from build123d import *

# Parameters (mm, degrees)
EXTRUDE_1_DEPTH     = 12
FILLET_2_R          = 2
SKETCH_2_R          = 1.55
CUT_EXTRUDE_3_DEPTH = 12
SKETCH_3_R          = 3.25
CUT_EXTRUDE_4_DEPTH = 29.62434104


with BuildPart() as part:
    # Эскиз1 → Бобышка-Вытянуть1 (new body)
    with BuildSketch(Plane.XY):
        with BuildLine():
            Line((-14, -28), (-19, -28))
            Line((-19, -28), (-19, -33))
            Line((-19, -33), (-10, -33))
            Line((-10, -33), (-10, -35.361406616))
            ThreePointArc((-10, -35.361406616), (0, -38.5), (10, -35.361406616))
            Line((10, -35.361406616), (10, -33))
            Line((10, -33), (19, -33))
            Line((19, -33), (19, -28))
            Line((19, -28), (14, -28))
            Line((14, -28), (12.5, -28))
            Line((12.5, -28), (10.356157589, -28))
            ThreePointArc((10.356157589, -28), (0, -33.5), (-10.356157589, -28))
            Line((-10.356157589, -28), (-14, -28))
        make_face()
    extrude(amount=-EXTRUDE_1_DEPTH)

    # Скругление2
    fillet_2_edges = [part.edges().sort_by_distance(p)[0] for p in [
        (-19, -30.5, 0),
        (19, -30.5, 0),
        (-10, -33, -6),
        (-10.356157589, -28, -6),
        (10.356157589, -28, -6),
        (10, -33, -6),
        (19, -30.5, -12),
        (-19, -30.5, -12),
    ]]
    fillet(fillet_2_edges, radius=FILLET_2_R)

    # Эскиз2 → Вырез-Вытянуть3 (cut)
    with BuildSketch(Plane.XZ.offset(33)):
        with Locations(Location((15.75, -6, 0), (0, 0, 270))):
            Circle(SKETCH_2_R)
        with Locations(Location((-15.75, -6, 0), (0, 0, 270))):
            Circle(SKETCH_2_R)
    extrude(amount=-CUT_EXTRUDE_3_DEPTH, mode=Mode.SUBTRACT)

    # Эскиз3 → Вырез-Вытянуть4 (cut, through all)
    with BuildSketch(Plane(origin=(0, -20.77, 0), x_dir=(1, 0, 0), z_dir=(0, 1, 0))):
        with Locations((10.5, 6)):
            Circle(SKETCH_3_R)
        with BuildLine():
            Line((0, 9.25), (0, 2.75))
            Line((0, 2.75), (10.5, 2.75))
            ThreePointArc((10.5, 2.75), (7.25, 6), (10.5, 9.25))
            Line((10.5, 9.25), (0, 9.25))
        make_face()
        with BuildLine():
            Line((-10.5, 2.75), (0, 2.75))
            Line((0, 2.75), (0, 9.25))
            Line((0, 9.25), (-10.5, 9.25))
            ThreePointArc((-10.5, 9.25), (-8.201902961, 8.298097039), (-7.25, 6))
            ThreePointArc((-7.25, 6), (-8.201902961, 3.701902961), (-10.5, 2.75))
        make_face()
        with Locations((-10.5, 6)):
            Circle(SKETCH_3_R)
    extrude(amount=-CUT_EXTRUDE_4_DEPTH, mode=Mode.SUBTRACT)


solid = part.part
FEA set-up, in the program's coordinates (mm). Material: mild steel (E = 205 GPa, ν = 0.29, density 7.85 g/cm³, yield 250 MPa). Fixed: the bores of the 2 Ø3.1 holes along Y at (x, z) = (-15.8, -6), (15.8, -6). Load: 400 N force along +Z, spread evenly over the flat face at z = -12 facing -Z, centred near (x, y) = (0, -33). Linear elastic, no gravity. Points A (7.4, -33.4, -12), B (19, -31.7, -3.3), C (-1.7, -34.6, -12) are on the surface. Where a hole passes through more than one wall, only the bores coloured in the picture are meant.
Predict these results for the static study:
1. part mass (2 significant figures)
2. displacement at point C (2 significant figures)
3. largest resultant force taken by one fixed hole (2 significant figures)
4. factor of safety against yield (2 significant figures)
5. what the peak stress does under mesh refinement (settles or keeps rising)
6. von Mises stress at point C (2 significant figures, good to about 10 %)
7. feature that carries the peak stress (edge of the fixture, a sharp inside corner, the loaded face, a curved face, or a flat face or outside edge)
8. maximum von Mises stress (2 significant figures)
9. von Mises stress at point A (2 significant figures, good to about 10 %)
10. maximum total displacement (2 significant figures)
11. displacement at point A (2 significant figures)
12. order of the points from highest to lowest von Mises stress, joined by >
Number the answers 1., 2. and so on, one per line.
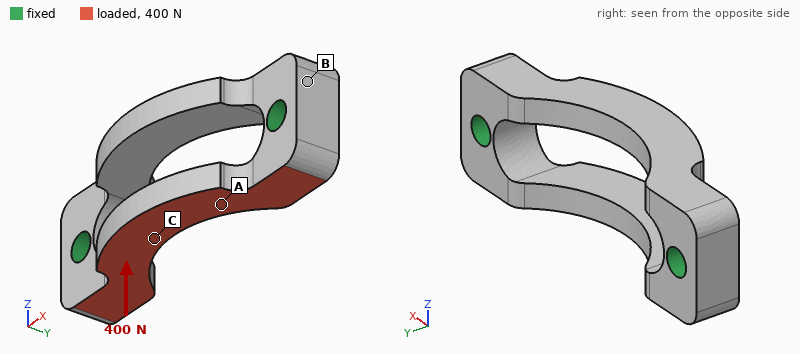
1. 11 g
2. 17 µm
3. 210 N
4. 1.2
5. settles
6. 67 MPa
7. a curved face
8. 220 MPa
9. 40 MPa
10. 24 µm
11. 10 µm
12. C > A > B
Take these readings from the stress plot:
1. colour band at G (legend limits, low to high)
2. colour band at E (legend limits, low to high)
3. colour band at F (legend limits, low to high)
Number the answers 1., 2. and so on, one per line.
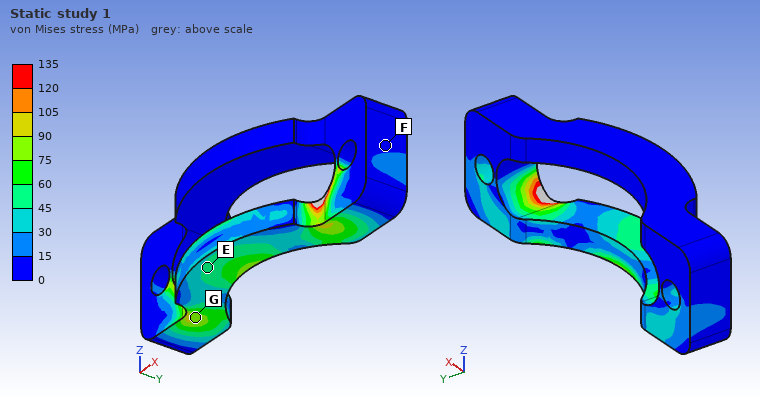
1. 75 to 90 MPa
2. 45 to 60 MPa
3. 0 to 15 MPa
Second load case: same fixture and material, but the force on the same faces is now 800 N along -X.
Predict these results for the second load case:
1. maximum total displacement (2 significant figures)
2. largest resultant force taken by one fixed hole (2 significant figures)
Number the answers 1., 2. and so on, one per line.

1. 3.4 µm
2. 410 N
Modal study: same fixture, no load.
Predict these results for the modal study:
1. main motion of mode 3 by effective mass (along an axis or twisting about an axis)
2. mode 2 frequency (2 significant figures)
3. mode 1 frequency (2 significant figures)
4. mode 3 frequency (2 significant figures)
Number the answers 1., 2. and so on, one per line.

1. twisting about X
2. 13 kHz
3. 13 kHz
4. 29 kHz
